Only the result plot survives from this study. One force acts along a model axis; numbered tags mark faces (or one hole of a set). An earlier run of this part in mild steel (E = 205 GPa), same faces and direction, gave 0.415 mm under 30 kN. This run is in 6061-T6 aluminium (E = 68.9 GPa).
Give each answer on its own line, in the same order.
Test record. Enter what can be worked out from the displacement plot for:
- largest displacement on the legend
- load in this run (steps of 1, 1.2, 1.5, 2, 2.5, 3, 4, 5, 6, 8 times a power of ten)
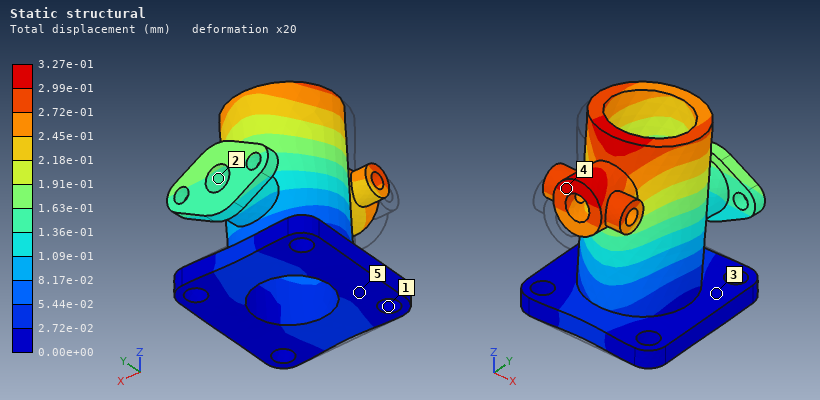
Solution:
3.27e-01 mm
8 kN
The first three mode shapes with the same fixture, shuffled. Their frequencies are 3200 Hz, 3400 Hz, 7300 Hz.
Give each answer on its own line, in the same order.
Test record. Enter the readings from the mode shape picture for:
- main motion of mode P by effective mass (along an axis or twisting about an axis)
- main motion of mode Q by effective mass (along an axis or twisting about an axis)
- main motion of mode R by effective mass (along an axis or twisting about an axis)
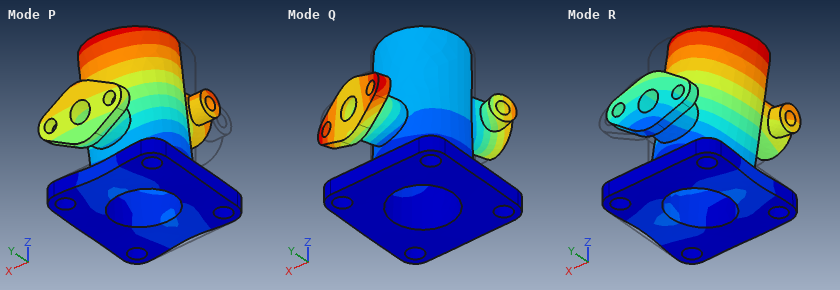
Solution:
along Y
twisting about Z
along X
